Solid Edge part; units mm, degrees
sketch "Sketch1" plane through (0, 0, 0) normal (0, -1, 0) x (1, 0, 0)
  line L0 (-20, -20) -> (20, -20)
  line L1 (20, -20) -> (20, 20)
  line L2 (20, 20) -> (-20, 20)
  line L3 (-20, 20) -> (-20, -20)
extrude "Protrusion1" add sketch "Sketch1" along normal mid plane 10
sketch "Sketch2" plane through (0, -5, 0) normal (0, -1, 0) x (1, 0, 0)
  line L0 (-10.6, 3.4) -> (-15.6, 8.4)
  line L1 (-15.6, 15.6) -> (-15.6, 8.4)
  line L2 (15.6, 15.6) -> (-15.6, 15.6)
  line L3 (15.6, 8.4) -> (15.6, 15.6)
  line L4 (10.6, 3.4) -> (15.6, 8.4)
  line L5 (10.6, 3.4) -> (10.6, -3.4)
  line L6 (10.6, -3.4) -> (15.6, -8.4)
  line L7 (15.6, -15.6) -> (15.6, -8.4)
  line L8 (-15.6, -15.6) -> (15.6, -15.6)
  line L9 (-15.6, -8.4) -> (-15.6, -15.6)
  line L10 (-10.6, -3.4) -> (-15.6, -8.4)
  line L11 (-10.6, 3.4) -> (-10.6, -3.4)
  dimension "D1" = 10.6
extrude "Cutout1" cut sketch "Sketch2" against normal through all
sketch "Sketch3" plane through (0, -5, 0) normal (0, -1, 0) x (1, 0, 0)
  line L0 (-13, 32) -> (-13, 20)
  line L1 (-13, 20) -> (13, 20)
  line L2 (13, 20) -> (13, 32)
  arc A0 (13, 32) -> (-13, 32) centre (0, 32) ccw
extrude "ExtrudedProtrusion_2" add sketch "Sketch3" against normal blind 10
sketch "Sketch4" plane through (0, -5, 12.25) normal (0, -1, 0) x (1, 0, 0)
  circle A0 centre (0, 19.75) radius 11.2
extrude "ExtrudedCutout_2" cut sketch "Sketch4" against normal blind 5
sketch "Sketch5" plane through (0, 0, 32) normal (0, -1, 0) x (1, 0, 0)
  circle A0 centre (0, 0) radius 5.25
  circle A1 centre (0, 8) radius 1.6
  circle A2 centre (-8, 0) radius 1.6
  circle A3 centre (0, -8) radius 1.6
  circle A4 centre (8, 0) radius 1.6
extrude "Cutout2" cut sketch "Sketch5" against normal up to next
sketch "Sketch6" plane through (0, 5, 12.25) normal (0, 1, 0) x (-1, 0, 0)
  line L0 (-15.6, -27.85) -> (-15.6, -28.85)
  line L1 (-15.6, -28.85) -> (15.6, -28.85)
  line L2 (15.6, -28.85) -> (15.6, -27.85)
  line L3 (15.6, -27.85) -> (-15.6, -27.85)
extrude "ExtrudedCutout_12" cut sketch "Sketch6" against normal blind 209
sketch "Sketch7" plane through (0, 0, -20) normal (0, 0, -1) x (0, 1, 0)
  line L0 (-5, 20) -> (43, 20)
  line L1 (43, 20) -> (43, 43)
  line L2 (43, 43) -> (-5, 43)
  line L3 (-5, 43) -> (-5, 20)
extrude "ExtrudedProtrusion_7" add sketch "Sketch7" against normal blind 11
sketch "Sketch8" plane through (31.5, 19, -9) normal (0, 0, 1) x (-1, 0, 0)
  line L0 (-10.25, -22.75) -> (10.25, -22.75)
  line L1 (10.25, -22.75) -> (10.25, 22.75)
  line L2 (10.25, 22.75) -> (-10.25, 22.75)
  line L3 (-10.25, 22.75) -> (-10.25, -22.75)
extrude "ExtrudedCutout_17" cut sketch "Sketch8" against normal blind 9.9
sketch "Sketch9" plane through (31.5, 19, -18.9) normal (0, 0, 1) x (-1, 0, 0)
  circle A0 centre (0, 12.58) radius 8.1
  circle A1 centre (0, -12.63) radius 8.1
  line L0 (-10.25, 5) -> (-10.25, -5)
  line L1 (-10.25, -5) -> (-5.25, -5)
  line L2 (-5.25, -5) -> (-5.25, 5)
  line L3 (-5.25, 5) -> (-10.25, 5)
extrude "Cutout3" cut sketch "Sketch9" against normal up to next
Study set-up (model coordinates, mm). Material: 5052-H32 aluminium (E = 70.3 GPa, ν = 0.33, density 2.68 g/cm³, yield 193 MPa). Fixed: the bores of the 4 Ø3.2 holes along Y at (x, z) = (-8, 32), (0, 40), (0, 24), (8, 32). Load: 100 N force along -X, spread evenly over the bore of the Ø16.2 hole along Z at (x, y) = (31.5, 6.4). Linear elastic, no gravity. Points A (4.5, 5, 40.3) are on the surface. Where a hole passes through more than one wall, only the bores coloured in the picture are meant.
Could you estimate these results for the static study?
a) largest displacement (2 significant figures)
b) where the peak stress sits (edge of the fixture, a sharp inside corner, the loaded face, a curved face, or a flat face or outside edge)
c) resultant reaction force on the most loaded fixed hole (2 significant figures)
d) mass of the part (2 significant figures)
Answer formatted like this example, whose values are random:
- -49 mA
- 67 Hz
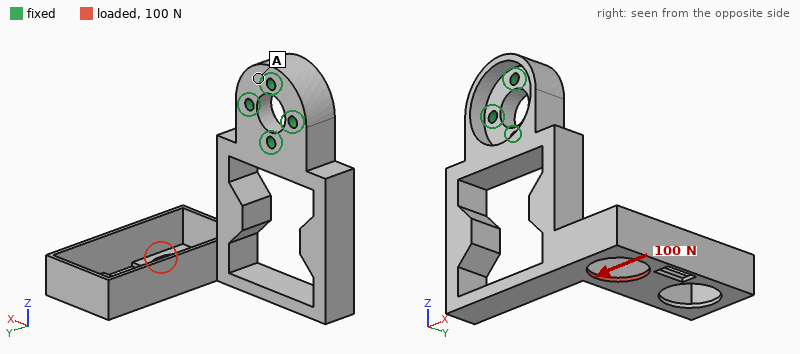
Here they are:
- 0.23 mm
- the loaded face
- 200 N
- 34 g
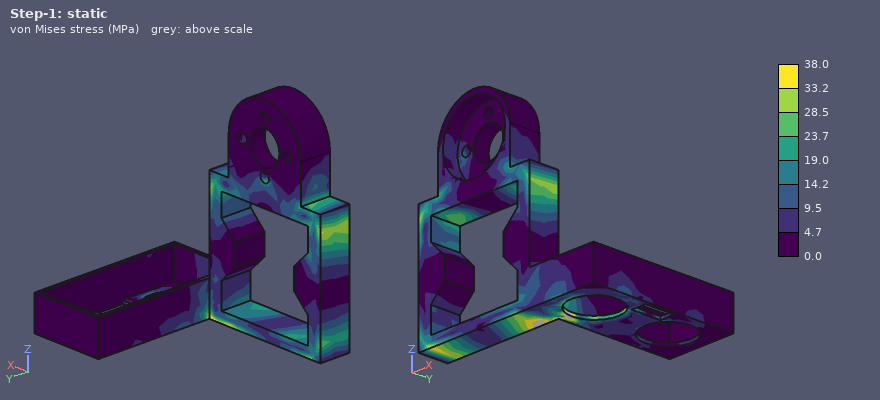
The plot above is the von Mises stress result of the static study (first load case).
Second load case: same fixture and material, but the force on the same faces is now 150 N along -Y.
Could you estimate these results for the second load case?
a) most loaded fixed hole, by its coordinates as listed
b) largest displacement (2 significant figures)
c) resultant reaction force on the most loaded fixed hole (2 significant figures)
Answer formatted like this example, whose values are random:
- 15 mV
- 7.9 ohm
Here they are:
- (0, 24)
- 0.70 mm
- 470 N
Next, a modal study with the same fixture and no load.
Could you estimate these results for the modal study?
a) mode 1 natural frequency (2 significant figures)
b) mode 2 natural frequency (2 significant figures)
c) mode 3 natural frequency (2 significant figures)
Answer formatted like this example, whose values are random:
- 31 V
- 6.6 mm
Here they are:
- 840 Hz
- 990 Hz
- 1300 Hz
